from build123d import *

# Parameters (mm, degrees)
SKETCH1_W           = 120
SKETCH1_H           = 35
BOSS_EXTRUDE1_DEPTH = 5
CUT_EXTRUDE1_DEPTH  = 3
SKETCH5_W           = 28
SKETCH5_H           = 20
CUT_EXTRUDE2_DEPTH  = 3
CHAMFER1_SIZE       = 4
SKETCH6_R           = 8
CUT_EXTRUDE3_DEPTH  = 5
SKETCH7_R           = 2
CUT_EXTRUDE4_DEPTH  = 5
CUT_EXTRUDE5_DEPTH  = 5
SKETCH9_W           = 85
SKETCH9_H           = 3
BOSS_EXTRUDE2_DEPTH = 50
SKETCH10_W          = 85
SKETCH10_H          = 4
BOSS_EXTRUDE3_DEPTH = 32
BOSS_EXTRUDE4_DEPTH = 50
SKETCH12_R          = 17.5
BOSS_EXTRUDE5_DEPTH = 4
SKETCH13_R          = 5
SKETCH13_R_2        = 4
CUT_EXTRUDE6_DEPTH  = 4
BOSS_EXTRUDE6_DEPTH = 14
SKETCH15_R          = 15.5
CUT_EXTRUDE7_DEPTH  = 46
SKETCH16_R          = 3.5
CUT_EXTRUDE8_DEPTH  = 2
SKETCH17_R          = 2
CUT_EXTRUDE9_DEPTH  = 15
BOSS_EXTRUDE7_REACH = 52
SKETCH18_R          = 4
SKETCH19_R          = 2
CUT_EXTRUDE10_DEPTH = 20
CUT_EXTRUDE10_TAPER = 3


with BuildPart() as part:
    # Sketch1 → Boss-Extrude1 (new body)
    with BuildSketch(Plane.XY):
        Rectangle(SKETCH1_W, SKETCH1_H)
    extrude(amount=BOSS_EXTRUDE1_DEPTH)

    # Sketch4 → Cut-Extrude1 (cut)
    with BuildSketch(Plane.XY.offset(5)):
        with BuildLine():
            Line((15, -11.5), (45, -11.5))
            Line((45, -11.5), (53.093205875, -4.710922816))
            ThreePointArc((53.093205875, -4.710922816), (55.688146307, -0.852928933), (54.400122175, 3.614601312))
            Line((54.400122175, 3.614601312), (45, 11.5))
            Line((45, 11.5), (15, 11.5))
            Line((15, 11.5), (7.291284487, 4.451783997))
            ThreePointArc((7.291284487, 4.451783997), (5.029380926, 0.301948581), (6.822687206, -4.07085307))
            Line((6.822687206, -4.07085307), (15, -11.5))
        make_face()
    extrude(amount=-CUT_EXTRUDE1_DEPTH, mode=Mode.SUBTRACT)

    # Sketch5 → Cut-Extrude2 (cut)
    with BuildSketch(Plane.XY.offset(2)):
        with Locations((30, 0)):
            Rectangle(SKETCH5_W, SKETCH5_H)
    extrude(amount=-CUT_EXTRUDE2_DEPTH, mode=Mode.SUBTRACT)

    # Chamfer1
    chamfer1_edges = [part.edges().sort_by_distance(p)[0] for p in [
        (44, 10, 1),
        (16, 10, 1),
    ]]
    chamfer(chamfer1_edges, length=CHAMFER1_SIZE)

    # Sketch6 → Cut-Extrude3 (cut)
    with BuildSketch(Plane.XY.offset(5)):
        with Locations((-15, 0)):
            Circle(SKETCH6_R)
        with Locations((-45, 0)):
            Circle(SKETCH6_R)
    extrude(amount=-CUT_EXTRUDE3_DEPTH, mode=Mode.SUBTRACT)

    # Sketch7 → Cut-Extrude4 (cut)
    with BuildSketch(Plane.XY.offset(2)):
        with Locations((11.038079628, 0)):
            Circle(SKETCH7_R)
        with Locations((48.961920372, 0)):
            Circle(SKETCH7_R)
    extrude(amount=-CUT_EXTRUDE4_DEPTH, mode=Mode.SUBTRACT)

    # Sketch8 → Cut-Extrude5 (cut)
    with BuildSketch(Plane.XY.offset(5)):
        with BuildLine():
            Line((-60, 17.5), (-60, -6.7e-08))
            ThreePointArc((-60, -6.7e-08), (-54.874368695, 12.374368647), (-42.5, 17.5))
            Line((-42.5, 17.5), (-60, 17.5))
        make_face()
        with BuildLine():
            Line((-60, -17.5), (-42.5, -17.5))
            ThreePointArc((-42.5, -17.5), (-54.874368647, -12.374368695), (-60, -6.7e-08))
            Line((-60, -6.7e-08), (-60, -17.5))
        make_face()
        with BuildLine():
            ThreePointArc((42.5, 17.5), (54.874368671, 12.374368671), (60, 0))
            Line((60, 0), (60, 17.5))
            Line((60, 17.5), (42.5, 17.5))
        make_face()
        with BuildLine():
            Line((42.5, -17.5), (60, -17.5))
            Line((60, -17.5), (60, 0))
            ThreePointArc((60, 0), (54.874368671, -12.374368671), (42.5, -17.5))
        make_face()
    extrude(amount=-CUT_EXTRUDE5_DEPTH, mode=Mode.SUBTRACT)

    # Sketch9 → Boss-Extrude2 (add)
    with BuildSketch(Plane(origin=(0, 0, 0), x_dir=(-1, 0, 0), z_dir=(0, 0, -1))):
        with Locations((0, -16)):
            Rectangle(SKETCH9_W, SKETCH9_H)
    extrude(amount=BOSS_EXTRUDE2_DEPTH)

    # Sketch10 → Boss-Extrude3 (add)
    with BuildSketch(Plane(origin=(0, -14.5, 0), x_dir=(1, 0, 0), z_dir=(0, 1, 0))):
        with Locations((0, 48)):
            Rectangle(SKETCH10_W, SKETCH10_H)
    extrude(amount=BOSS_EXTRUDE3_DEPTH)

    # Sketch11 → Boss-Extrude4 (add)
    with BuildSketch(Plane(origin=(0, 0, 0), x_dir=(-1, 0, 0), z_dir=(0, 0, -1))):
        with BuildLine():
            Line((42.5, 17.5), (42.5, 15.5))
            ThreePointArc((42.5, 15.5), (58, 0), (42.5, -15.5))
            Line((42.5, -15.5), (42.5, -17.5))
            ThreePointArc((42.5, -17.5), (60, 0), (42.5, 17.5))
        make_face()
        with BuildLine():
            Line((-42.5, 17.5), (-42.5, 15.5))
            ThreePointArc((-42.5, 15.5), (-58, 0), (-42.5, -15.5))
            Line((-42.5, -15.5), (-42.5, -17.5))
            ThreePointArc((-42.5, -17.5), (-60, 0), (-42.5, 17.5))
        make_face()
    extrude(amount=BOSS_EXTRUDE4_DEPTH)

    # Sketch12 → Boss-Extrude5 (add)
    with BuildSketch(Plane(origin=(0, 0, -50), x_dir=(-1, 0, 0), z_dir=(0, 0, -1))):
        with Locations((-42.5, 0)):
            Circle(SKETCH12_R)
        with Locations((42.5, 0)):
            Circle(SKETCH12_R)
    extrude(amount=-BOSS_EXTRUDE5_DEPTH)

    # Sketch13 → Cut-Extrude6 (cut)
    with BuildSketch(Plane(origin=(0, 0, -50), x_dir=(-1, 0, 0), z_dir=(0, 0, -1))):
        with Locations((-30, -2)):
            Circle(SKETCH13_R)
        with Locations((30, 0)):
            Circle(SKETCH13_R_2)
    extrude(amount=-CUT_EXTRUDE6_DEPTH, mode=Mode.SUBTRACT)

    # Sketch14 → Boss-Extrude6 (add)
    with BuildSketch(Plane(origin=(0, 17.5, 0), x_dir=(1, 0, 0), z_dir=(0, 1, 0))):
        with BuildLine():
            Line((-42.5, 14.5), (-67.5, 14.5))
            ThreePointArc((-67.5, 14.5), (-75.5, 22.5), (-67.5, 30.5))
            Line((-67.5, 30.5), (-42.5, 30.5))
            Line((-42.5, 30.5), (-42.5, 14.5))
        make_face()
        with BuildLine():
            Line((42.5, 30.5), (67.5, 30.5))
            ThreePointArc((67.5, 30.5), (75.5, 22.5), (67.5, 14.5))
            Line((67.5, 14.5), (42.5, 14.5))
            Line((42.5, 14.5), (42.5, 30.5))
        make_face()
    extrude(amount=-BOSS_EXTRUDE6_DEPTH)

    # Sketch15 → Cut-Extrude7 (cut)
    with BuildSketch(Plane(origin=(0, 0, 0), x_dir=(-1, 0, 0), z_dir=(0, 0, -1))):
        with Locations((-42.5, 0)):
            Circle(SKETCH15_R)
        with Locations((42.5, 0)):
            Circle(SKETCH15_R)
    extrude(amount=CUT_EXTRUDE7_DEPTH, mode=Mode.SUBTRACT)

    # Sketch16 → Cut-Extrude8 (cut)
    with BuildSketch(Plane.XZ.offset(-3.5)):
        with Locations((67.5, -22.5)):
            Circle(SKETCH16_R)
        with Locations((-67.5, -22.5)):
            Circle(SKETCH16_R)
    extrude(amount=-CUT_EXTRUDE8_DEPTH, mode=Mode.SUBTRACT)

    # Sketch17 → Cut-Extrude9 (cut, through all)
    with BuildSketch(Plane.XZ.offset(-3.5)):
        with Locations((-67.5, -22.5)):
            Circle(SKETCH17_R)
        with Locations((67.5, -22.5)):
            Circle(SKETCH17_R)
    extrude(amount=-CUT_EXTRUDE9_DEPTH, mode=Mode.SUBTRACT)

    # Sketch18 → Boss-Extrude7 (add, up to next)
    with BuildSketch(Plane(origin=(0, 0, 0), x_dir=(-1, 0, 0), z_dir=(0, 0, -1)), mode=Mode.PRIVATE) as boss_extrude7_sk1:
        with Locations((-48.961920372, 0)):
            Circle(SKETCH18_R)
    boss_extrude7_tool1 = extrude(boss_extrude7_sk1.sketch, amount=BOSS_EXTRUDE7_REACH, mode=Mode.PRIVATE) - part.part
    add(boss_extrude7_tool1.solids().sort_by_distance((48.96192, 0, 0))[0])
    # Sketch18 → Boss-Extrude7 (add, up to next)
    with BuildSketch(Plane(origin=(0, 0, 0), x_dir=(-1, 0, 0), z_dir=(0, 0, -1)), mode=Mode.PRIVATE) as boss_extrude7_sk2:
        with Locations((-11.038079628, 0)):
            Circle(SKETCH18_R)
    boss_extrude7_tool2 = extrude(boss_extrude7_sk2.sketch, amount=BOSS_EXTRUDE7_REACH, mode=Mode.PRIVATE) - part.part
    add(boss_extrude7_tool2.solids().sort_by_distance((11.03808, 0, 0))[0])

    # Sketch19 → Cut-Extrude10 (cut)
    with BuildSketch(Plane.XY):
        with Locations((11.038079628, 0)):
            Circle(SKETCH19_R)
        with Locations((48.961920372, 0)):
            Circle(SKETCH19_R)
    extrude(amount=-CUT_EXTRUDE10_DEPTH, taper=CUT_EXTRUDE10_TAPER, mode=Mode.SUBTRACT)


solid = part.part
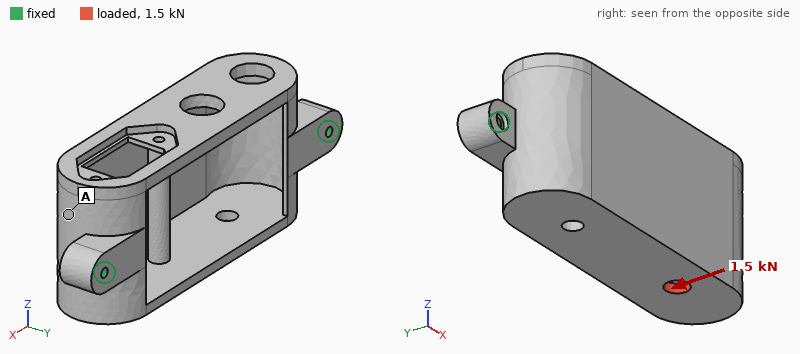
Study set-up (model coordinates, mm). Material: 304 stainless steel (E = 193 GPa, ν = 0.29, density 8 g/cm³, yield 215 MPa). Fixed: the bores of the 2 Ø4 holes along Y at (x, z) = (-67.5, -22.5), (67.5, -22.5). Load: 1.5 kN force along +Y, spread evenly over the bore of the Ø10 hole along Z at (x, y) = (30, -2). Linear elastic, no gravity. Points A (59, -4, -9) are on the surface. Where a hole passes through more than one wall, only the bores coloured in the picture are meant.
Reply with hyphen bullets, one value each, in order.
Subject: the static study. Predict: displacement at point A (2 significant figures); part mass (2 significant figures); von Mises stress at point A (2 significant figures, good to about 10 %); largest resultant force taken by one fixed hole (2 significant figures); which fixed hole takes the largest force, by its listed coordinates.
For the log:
- 15 µm
- 500 g
- 11 MPa
- 1.1 kN
- (67.5, -22.5)
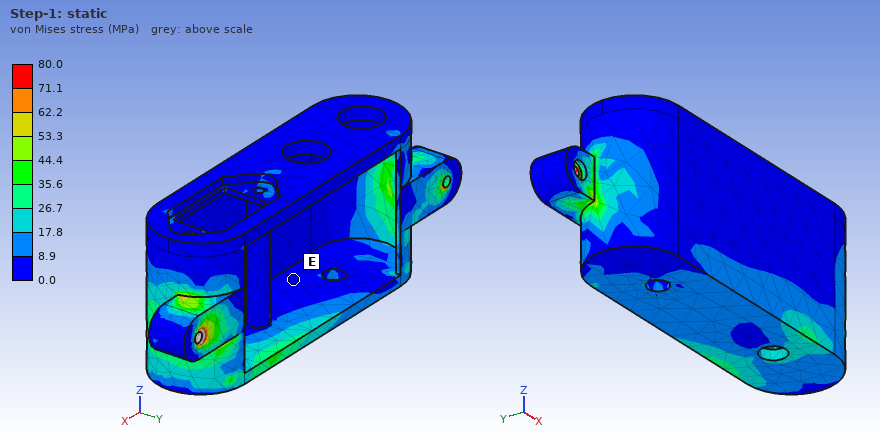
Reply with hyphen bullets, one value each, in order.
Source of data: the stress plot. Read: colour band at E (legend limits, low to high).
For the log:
- 0.0 to 8.9 MPa
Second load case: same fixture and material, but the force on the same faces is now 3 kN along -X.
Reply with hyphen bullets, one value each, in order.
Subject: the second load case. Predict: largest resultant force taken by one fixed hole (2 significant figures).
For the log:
- 1.6 kN
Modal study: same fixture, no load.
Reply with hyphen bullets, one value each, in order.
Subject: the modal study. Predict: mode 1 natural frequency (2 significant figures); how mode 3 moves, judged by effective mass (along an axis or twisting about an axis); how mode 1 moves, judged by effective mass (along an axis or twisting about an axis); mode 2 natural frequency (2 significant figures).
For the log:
- 1900 Hz
- along X
- along Z
- 2700 Hz
